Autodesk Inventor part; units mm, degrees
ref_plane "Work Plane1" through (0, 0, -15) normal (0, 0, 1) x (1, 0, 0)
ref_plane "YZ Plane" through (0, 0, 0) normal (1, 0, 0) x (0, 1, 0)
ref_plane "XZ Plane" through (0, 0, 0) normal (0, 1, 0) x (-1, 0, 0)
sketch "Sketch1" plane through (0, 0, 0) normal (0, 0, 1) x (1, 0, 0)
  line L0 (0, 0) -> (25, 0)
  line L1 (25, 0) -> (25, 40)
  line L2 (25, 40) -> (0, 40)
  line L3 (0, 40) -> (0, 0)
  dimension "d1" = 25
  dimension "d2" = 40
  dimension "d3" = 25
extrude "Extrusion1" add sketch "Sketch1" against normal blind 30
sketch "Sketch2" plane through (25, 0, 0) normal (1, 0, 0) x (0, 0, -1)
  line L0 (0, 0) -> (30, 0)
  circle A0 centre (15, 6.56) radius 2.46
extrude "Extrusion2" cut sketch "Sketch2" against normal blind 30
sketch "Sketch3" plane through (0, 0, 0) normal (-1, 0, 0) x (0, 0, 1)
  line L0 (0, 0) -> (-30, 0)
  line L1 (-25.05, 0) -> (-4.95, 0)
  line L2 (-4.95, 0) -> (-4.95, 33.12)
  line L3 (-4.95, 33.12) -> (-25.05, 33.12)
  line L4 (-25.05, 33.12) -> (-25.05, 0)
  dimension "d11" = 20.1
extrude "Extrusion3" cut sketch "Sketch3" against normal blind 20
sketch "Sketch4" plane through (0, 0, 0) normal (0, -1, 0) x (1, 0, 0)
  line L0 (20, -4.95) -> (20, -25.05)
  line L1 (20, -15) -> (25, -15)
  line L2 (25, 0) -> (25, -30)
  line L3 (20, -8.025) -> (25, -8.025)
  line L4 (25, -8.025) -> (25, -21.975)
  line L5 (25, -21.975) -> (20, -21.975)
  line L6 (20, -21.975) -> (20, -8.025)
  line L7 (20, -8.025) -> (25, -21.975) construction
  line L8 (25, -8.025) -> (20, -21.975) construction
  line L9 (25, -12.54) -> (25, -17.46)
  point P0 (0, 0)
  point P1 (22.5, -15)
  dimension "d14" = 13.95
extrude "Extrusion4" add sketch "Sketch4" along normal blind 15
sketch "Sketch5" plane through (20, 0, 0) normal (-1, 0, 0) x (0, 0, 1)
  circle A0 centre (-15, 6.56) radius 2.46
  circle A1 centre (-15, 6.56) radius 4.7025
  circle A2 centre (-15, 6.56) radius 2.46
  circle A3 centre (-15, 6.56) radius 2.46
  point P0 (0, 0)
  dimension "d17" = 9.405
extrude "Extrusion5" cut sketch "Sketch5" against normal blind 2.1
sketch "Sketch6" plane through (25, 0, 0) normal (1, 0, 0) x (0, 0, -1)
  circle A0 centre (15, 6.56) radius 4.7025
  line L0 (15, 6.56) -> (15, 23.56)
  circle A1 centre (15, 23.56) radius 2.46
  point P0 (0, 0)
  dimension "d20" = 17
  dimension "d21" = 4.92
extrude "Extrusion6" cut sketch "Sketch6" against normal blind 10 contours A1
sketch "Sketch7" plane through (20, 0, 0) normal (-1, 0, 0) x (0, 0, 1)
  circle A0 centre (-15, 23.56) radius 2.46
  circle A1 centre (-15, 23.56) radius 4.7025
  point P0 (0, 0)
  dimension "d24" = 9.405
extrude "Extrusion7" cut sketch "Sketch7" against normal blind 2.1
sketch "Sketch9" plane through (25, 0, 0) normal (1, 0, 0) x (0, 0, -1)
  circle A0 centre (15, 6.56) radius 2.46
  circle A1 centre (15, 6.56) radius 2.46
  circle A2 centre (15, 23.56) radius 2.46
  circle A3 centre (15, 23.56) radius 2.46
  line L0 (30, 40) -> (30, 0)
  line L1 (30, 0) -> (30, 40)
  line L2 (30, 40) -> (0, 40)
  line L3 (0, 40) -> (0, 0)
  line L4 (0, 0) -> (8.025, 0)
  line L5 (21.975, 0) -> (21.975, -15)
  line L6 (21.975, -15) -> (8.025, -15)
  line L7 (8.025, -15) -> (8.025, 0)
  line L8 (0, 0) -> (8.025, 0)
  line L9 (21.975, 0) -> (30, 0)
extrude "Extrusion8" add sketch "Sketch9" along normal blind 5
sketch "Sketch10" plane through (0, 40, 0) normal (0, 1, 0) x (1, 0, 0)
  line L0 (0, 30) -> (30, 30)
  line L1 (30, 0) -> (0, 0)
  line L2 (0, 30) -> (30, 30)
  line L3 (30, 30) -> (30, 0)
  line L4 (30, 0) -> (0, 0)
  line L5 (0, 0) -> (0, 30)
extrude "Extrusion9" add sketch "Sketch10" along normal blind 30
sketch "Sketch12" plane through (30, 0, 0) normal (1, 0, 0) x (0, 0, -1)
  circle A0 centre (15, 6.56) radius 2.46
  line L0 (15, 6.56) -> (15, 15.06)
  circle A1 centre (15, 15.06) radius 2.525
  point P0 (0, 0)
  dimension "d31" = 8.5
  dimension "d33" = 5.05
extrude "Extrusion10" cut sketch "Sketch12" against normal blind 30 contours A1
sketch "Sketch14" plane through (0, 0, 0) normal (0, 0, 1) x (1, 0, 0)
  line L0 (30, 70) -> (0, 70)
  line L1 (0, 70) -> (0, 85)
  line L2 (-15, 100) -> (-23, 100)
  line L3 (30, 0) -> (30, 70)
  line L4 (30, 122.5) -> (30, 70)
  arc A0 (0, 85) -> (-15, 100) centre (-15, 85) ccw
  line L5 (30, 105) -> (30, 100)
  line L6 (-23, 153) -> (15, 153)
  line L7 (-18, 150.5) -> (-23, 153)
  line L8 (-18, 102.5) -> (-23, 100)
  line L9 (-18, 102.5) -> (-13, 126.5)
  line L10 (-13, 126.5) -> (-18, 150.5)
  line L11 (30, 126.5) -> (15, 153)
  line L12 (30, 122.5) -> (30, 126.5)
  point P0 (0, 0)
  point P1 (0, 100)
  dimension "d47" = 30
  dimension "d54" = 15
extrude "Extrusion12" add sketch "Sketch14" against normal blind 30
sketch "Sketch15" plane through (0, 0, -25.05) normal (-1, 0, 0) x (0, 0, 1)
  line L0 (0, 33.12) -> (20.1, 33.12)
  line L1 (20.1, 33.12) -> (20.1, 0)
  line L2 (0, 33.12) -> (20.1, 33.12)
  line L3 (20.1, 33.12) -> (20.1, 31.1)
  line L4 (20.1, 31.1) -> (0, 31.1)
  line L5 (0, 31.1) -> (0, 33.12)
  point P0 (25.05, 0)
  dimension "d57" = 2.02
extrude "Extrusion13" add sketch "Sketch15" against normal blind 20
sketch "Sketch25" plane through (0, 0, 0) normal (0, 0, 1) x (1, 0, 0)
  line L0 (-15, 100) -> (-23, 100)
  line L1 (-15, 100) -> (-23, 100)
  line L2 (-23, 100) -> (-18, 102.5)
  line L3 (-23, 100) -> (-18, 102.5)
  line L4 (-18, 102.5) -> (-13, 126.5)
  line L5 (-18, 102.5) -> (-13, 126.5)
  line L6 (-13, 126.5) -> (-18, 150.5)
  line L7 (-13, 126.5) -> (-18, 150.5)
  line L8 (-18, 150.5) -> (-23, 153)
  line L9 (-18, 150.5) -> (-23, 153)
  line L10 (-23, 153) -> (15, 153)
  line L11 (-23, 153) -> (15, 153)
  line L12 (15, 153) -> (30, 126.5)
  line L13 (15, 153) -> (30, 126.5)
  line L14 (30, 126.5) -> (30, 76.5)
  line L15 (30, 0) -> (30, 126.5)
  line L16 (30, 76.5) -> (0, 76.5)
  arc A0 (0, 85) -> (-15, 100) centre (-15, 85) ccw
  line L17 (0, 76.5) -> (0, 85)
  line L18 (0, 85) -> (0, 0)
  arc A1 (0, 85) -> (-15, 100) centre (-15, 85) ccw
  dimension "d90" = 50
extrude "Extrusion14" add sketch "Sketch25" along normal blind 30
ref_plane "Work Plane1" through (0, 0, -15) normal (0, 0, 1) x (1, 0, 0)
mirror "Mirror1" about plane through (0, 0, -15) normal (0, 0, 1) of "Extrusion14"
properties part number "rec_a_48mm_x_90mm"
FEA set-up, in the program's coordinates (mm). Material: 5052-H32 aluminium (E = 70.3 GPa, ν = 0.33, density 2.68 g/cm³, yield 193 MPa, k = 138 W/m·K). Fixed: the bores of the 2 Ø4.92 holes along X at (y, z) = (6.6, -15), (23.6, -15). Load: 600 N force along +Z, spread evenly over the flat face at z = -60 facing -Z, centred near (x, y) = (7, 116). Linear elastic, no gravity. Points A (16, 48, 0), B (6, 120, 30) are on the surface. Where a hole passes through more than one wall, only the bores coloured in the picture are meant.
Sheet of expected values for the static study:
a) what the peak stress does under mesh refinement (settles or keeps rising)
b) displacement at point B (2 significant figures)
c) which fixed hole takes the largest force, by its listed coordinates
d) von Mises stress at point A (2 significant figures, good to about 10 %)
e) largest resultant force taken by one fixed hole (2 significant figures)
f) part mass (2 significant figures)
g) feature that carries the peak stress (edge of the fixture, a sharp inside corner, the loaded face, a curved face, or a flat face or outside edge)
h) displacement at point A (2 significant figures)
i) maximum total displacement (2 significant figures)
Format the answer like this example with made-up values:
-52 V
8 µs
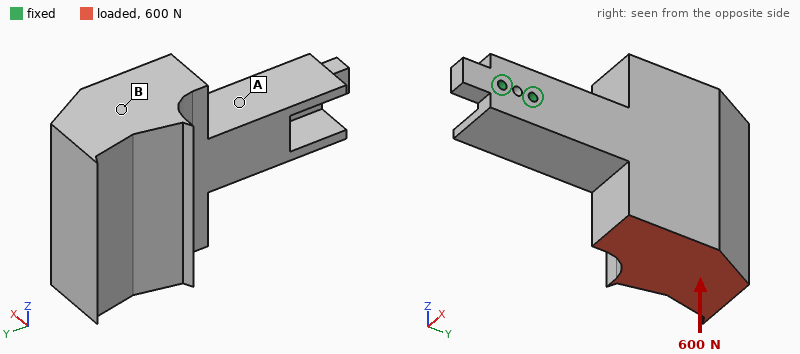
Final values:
keeps rising
0.12 mm
(23.6, -15)
9.6 MPa
3.0 kN
880 g
edge of the fixture
0.029 mm
0.17 mm
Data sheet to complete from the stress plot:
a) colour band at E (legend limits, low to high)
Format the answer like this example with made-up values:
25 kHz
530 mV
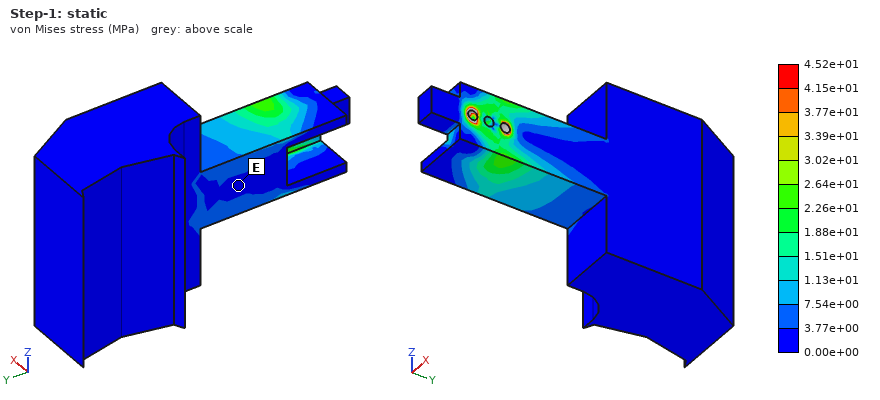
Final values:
0.00e+00 to 3.77e+00 MPa
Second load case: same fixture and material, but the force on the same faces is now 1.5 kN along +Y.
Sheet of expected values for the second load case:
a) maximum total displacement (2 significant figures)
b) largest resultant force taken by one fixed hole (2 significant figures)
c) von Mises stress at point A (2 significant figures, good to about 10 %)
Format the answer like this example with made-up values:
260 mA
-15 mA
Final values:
0.25 mm
3.2 kN
14 MPa
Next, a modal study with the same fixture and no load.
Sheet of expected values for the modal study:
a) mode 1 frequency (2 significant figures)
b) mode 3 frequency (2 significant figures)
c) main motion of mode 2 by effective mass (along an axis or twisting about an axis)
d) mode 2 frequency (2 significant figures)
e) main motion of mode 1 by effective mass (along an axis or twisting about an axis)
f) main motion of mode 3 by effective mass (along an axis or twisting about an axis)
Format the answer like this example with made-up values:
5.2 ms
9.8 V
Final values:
370 Hz
810 Hz
along Z
410 Hz
along X
twisting about Y
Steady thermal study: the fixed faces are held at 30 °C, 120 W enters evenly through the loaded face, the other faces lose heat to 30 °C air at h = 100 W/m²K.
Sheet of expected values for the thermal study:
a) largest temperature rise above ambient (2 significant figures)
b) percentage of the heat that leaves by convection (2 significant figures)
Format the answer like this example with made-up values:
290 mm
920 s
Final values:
41 K
72 %
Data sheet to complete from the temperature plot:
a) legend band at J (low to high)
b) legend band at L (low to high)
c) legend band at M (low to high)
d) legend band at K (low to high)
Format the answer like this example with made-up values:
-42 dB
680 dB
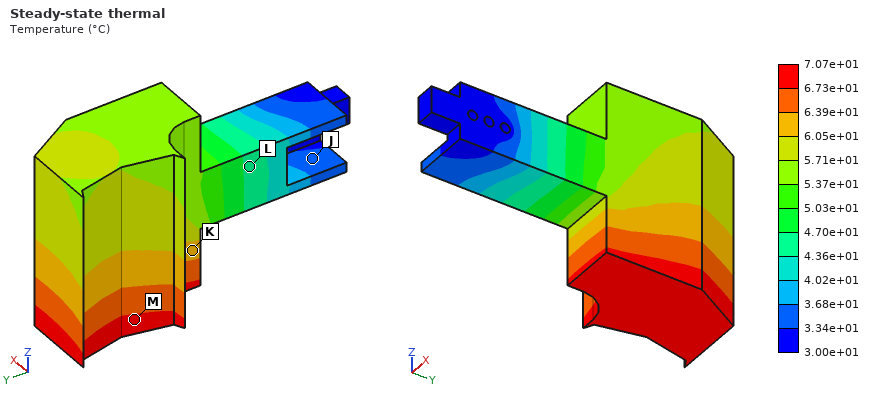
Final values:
3.34e+01 to 3.68e+01 °C
4.36e+01 to 4.70e+01 °C
6.73e+01 to 7.07e+01 °C
6.05e+01 to 6.39e+01 °C
